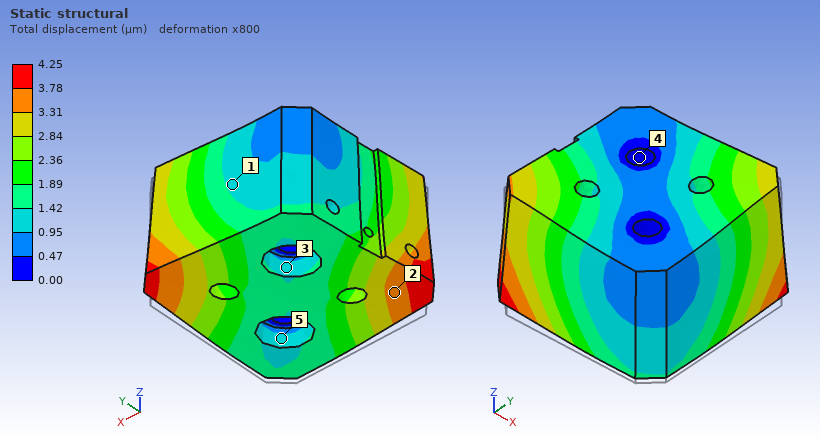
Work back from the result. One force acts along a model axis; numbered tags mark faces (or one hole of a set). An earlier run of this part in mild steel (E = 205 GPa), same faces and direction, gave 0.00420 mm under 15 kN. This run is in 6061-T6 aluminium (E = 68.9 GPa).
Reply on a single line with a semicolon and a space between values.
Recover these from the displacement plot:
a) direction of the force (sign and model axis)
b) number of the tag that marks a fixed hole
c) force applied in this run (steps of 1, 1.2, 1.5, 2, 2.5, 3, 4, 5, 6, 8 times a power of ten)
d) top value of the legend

+Z; 4; 5 kN; 4.25 µm
